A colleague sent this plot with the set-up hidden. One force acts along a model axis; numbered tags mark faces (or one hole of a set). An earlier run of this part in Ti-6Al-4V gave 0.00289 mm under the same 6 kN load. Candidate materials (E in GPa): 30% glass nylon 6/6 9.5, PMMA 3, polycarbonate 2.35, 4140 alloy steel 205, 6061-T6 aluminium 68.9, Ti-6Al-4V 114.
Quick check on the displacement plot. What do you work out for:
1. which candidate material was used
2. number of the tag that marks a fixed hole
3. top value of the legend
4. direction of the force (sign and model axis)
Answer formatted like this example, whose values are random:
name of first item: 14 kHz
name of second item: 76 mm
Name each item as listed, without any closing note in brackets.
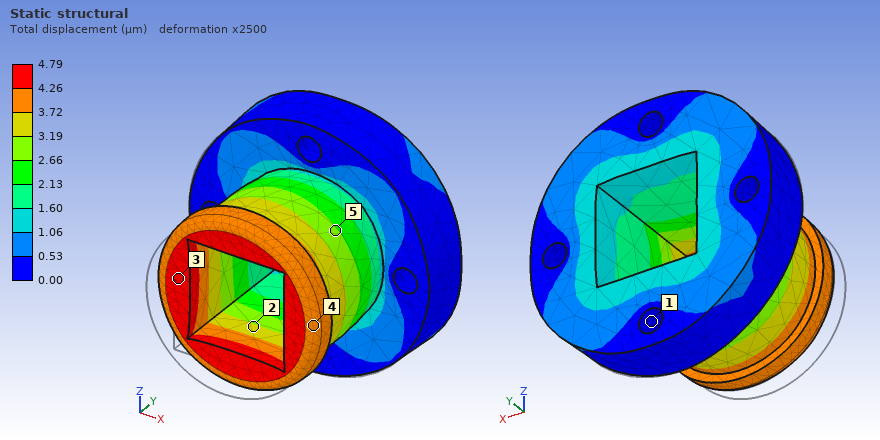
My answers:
which candidate material was used: 6061-T6 aluminium
number of the tag that marks a fixed hole: 1
top value of the legend: 4.79 µm
direction of the force: +Y
